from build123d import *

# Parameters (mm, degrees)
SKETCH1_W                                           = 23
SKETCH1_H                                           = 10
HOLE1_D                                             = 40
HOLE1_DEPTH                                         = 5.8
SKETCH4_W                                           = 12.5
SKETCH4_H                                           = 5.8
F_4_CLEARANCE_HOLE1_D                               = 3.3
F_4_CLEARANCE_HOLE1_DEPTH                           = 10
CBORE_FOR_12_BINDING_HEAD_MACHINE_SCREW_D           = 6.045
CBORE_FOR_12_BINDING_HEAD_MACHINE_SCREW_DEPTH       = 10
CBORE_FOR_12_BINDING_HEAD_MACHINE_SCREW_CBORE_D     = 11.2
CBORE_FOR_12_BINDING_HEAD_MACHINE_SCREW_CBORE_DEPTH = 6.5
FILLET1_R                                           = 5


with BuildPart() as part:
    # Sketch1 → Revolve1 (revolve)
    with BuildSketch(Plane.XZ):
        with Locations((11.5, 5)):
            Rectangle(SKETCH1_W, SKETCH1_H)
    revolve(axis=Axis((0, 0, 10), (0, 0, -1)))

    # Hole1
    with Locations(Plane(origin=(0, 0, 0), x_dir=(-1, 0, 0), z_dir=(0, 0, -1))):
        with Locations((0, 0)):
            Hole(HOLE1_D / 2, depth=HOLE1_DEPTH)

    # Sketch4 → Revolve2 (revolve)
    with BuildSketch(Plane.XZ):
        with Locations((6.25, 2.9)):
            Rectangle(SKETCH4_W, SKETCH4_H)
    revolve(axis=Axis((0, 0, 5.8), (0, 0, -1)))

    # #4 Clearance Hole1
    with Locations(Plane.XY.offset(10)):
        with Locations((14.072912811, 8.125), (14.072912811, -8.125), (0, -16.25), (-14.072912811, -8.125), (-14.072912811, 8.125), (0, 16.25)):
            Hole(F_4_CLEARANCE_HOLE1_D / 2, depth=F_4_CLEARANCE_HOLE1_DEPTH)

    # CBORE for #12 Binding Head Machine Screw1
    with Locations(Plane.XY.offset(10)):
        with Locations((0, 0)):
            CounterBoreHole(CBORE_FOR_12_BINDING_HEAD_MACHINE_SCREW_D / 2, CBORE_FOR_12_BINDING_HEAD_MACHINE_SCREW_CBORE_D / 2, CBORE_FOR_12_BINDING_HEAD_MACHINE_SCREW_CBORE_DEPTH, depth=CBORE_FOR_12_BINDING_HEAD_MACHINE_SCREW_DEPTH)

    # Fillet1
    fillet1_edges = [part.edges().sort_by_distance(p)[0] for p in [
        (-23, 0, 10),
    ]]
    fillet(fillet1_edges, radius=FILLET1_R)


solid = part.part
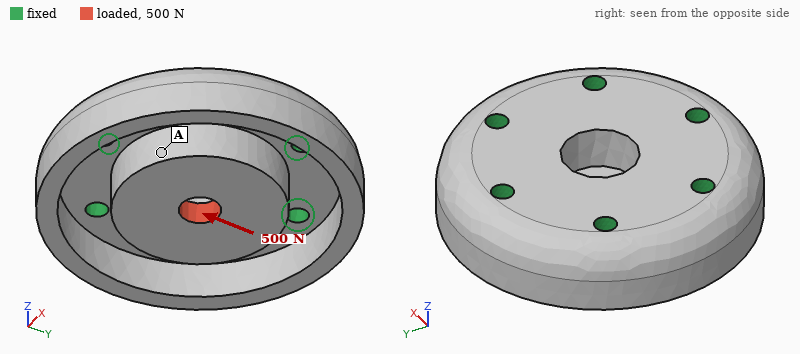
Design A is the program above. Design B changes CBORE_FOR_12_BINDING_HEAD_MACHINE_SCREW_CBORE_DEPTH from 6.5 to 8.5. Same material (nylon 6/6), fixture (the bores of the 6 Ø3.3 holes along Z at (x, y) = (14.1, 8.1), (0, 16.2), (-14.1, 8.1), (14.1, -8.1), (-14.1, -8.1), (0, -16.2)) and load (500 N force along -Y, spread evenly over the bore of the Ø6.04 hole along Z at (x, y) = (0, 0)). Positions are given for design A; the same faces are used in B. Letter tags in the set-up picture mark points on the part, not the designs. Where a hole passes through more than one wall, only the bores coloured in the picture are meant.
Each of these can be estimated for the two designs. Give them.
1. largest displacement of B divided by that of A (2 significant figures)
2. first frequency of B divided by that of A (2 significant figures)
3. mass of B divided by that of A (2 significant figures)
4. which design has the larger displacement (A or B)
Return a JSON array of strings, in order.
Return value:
["1.7", "1.00", "0.99", "B"]
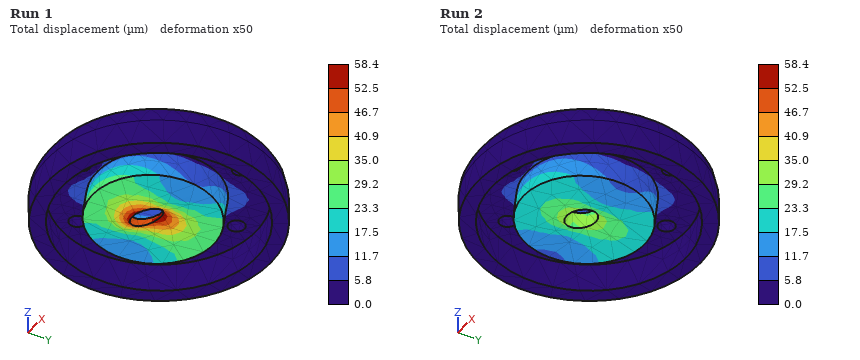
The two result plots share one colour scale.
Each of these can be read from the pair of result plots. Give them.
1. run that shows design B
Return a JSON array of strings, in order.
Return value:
["Run 1"]
